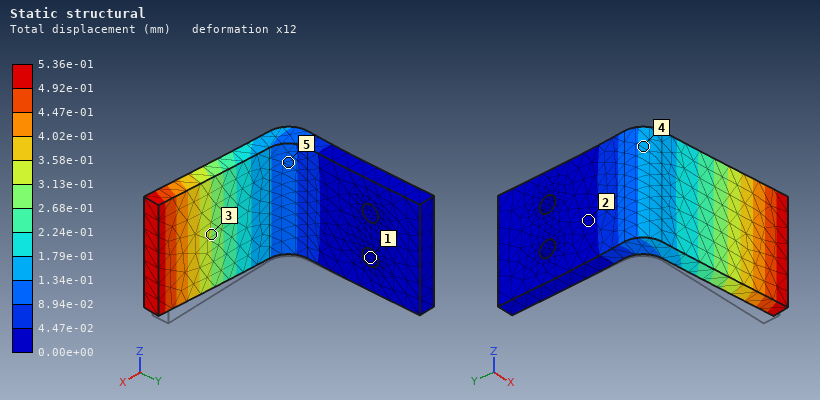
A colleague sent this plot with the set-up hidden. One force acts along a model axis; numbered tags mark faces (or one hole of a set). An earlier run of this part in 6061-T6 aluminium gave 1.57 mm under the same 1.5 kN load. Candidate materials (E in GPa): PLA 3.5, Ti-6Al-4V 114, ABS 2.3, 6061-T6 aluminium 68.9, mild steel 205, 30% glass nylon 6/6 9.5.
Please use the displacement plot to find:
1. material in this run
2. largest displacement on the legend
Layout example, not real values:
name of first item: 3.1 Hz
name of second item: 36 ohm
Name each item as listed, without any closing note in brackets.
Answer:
material in this run: mild steel
largest displacement on the legend: 5.36e-01 mm
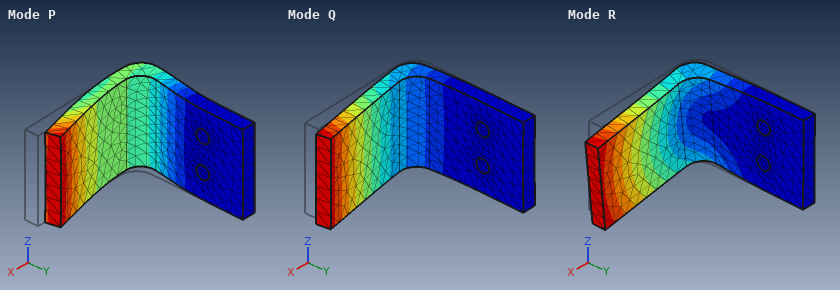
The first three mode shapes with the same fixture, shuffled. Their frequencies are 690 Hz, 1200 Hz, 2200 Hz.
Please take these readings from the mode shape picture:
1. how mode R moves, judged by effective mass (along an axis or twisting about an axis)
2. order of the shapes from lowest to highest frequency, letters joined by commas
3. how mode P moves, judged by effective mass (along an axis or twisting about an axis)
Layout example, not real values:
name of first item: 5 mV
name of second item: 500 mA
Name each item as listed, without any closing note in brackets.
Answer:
how mode R moves, judged by effective mass: along Z
order of the shapes from lowest to highest frequency, letters joined by commas: Q, R, P
how mode P moves, judged by effective mass: along X
